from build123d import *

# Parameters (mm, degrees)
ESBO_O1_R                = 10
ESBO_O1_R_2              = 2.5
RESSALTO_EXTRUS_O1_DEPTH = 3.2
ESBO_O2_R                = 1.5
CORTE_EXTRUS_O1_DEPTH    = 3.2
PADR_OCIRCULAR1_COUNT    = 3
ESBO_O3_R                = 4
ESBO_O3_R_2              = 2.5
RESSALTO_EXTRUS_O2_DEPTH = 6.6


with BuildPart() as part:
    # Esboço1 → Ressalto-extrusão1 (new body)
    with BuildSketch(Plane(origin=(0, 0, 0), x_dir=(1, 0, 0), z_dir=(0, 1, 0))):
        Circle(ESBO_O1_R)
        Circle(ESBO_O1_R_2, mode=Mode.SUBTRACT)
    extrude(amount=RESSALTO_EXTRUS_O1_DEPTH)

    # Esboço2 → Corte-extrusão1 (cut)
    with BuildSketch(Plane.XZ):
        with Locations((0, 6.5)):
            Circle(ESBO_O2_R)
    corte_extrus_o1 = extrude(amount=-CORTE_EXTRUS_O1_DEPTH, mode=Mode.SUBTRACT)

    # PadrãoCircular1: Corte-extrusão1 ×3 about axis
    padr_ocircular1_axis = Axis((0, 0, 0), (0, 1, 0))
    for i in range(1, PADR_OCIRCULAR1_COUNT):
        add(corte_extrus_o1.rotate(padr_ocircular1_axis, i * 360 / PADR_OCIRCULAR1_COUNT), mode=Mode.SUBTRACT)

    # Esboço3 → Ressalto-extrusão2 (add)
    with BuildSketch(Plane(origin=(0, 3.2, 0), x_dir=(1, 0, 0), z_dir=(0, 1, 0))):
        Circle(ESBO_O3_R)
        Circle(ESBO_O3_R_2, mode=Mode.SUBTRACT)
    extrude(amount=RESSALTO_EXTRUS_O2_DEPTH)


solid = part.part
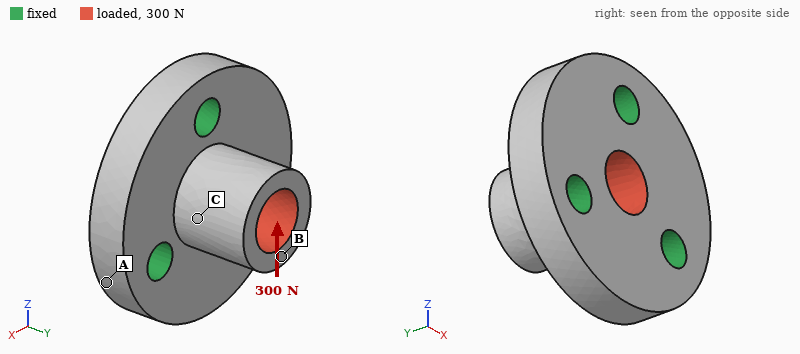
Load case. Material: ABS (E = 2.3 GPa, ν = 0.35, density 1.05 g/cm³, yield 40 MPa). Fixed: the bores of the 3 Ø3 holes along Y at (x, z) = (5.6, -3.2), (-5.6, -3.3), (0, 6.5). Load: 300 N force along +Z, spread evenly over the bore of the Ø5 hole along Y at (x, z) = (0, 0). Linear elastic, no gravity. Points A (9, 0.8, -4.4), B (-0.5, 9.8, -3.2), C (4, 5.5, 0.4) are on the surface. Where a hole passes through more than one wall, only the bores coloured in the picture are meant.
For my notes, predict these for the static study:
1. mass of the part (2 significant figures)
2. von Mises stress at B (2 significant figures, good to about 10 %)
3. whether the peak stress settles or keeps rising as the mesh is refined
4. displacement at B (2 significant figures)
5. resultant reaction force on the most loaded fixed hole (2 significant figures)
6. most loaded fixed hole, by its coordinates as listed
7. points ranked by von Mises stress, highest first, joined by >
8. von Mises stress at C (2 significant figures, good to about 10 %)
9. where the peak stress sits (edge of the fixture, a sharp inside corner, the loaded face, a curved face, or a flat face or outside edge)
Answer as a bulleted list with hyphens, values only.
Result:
- 1.1 g
- 6.2 MPa
- keeps rising
- 0.12 mm
- 150 N
- (0, 6.5)
- C > B > A
- 10 MPa
- a sharp inside corner
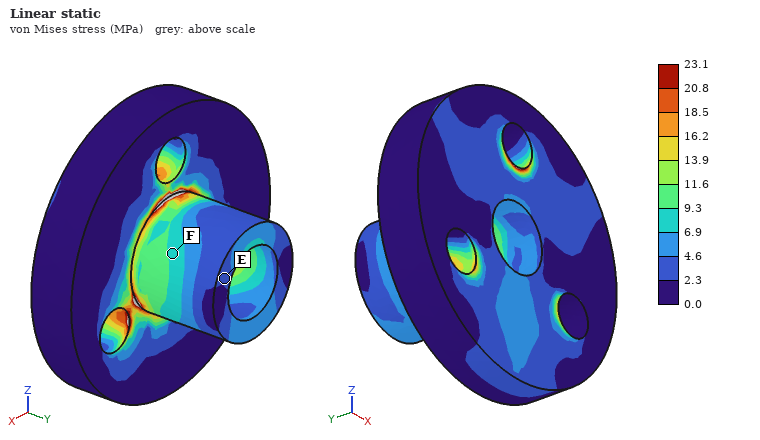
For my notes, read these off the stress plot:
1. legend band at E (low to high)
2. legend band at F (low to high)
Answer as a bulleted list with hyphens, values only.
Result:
- 2.3 to 4.6 MPa
- 6.9 to 9.3 MPa
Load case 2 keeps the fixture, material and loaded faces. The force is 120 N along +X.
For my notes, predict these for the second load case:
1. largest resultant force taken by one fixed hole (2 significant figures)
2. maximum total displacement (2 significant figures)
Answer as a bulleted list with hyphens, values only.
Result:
- 54 N
- 47 µm
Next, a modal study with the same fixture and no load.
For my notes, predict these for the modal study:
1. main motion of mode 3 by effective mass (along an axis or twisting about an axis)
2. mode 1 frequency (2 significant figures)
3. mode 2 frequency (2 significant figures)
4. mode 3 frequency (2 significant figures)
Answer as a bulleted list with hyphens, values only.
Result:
- along Y
- 16 kHz
- 16 kHz
- 19 kHz
